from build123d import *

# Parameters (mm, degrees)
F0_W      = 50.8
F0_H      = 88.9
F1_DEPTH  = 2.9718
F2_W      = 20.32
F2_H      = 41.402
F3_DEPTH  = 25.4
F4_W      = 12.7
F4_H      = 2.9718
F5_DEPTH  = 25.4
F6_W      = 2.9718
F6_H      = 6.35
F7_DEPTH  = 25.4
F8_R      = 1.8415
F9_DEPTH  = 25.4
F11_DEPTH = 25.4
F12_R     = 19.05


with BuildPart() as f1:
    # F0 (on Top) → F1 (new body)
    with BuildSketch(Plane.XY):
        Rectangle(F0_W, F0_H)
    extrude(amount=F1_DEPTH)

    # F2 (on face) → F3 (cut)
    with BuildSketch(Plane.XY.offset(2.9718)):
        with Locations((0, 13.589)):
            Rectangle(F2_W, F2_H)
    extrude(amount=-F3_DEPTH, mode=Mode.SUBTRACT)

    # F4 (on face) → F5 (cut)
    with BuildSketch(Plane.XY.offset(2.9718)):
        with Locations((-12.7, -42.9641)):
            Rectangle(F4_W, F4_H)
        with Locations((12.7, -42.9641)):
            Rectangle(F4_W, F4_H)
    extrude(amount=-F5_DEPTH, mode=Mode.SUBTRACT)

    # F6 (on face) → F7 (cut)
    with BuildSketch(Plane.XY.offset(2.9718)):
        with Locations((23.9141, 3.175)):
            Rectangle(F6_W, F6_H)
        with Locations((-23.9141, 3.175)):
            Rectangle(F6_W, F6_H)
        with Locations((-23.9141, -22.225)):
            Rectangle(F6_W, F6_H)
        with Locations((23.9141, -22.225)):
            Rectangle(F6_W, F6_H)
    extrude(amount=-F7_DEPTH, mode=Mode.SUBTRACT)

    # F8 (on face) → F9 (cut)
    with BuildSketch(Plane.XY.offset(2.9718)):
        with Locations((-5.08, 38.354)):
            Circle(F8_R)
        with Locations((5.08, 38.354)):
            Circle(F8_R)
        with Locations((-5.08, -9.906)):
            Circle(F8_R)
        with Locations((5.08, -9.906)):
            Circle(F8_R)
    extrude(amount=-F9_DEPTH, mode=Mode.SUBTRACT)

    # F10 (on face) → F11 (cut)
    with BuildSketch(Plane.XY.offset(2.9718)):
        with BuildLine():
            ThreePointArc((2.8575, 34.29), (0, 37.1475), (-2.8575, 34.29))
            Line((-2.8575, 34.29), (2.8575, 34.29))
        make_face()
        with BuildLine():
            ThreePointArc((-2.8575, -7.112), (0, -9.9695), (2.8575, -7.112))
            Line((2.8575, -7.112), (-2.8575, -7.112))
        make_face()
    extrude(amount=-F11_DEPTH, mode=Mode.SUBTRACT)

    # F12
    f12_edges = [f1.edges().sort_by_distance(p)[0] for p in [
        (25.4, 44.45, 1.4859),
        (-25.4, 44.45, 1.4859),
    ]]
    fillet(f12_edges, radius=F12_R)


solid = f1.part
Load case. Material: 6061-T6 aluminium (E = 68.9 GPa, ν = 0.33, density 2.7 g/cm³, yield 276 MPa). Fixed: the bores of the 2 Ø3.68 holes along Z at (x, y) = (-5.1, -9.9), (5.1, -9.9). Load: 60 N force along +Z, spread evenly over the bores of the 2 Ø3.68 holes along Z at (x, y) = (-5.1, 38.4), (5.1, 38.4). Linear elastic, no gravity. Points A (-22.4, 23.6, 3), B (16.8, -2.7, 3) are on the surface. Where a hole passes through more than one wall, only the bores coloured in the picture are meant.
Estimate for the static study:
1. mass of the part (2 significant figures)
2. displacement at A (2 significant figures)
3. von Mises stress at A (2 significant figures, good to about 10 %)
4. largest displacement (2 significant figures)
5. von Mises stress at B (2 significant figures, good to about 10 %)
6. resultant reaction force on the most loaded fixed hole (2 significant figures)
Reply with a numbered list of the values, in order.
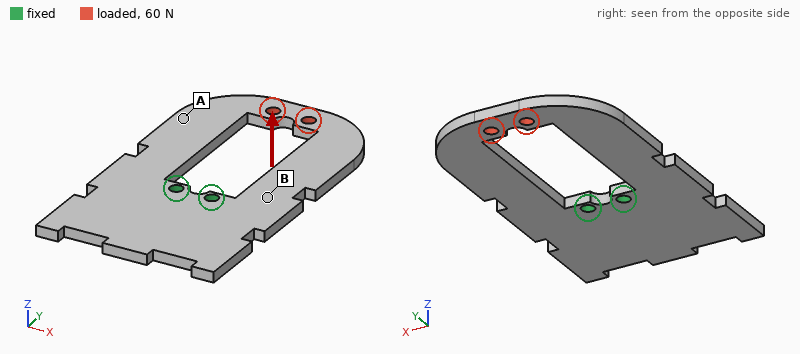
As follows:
1. 26 g
2. 0.45 mm
3. 20 MPa
4. 0.90 mm
5. 62 MPa
6. 30 N
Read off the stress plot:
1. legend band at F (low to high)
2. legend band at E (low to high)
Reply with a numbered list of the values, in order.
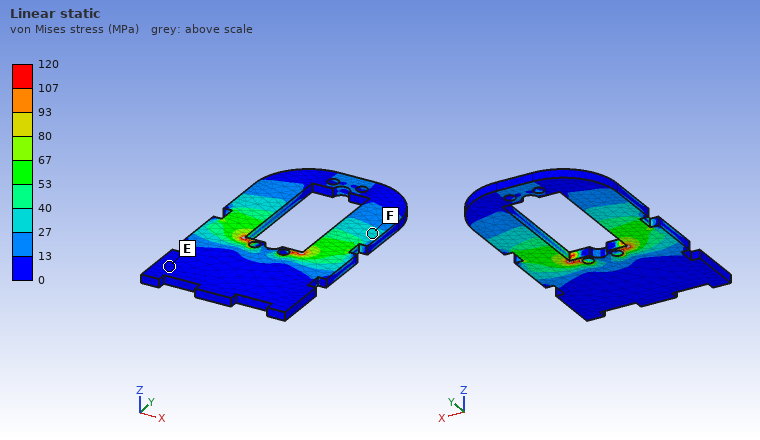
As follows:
1. 27 to 40 MPa
2. 0 to 13 MPa
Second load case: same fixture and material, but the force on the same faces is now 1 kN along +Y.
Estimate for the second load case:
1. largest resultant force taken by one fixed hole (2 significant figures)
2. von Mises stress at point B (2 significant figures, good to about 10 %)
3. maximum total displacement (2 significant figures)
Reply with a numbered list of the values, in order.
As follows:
1. 580 N
2. 12 MPa
3. 43 µm
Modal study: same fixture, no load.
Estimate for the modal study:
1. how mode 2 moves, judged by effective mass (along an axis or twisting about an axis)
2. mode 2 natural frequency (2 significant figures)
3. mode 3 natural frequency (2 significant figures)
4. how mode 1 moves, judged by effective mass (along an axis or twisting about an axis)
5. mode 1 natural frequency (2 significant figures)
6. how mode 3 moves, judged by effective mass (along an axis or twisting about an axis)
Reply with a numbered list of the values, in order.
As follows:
1. twisting about Y
2. 1500 Hz
3. 2000 Hz
4. along Z
5. 630 Hz
6. along Z
